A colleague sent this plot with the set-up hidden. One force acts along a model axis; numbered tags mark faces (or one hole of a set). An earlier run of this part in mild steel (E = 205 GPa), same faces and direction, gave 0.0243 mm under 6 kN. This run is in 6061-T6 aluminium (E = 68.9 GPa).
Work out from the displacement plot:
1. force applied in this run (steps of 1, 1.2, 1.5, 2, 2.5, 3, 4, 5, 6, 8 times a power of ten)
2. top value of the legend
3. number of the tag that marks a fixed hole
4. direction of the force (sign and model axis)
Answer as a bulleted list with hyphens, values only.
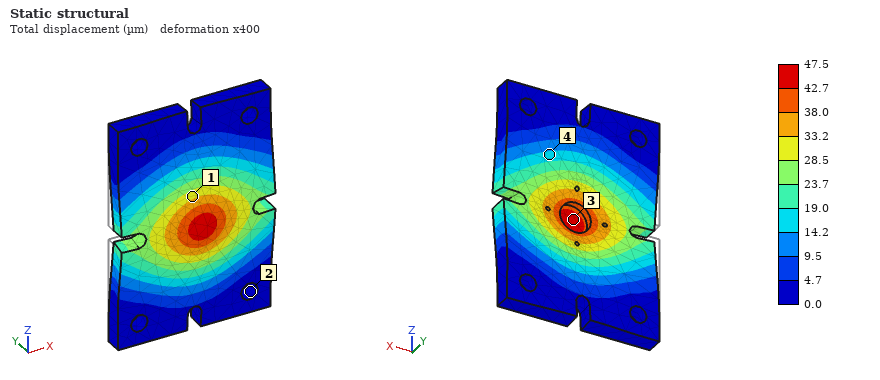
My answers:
- 4 kN
- 47.5 µm
- 2
- -Y
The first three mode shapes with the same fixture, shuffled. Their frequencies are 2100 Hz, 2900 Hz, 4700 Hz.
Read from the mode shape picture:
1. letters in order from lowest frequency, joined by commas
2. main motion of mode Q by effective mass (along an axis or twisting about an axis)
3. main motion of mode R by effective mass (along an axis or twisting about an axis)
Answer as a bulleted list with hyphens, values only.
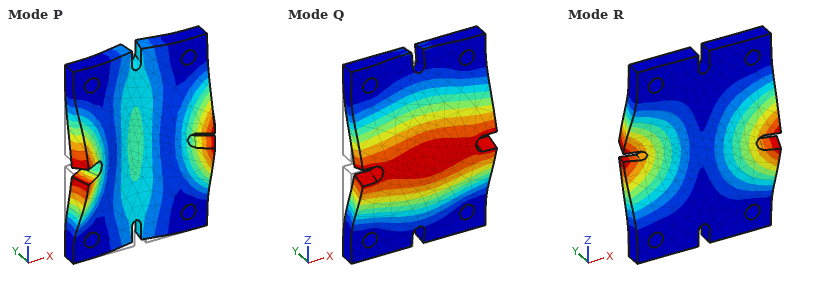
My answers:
- Q, R, P
- along Y
- twisting about Z
